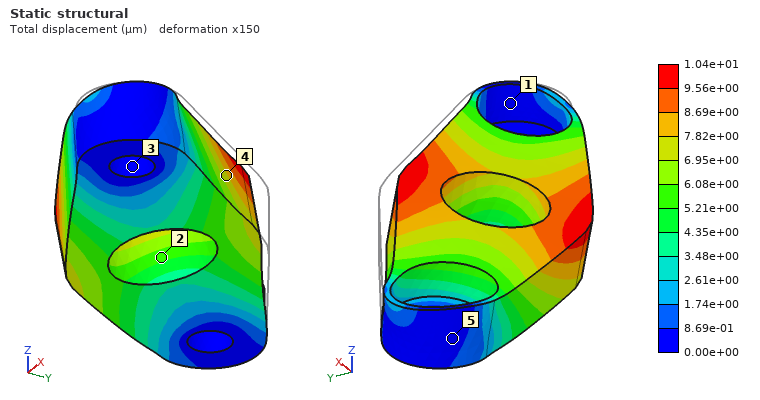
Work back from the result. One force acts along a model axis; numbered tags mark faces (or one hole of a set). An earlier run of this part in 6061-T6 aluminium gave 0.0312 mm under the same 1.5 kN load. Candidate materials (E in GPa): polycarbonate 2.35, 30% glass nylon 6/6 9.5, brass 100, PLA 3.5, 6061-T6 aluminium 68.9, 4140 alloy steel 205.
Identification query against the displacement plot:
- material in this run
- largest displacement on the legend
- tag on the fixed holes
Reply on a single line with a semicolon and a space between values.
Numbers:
4140 alloy steel; 1.04e+01 µm; 3
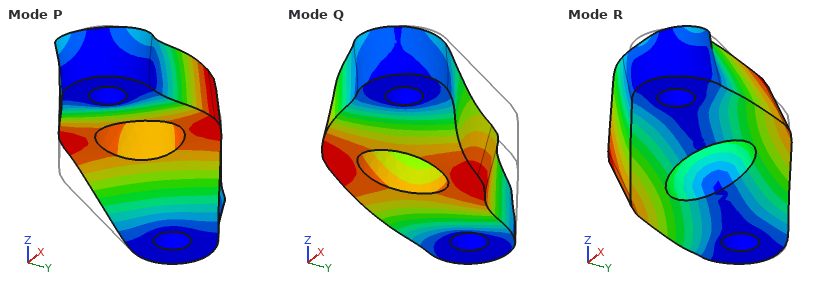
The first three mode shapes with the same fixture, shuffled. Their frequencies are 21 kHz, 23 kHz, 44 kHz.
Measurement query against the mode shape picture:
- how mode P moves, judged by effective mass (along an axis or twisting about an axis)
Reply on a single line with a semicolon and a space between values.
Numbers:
along Z
